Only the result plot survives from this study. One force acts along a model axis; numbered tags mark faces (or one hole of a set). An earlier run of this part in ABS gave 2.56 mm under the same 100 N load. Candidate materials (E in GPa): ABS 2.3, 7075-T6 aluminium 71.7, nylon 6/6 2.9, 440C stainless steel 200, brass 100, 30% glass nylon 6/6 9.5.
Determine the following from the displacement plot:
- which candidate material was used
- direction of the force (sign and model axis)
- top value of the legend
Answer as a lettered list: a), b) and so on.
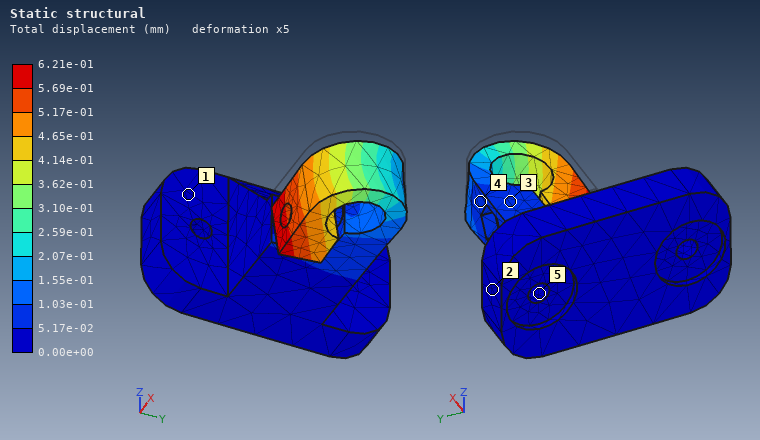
a) 30% glass nylon 6/6
b) -Z
c) 6.21e-01 mm
